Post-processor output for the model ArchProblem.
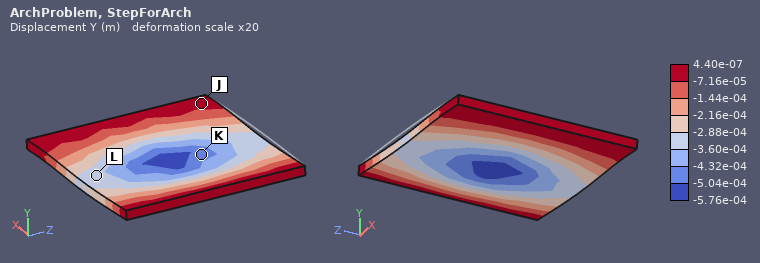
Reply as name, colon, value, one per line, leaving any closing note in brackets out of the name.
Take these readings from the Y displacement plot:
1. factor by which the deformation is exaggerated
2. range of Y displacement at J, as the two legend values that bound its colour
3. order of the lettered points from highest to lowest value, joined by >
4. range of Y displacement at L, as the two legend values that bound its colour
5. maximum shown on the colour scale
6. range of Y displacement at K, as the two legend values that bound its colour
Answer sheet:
factor by which the deformation is exaggerated: 20
range of Y displacement at J, as the two legend values that bound its colour: -7.16e-05 to 4.40e-07 m
order of the lettered points from highest to lowest value, joined by >: J > L > K
range of Y displacement at L, as the two legend values that bound its colour: -3.60e-04 to -2.88e-04 m
maximum shown on the colour scale: 4.40e-07 m
range of Y displacement at K, as the two legend values that bound its colour: -5.04e-04 to -4.32e-04 m
